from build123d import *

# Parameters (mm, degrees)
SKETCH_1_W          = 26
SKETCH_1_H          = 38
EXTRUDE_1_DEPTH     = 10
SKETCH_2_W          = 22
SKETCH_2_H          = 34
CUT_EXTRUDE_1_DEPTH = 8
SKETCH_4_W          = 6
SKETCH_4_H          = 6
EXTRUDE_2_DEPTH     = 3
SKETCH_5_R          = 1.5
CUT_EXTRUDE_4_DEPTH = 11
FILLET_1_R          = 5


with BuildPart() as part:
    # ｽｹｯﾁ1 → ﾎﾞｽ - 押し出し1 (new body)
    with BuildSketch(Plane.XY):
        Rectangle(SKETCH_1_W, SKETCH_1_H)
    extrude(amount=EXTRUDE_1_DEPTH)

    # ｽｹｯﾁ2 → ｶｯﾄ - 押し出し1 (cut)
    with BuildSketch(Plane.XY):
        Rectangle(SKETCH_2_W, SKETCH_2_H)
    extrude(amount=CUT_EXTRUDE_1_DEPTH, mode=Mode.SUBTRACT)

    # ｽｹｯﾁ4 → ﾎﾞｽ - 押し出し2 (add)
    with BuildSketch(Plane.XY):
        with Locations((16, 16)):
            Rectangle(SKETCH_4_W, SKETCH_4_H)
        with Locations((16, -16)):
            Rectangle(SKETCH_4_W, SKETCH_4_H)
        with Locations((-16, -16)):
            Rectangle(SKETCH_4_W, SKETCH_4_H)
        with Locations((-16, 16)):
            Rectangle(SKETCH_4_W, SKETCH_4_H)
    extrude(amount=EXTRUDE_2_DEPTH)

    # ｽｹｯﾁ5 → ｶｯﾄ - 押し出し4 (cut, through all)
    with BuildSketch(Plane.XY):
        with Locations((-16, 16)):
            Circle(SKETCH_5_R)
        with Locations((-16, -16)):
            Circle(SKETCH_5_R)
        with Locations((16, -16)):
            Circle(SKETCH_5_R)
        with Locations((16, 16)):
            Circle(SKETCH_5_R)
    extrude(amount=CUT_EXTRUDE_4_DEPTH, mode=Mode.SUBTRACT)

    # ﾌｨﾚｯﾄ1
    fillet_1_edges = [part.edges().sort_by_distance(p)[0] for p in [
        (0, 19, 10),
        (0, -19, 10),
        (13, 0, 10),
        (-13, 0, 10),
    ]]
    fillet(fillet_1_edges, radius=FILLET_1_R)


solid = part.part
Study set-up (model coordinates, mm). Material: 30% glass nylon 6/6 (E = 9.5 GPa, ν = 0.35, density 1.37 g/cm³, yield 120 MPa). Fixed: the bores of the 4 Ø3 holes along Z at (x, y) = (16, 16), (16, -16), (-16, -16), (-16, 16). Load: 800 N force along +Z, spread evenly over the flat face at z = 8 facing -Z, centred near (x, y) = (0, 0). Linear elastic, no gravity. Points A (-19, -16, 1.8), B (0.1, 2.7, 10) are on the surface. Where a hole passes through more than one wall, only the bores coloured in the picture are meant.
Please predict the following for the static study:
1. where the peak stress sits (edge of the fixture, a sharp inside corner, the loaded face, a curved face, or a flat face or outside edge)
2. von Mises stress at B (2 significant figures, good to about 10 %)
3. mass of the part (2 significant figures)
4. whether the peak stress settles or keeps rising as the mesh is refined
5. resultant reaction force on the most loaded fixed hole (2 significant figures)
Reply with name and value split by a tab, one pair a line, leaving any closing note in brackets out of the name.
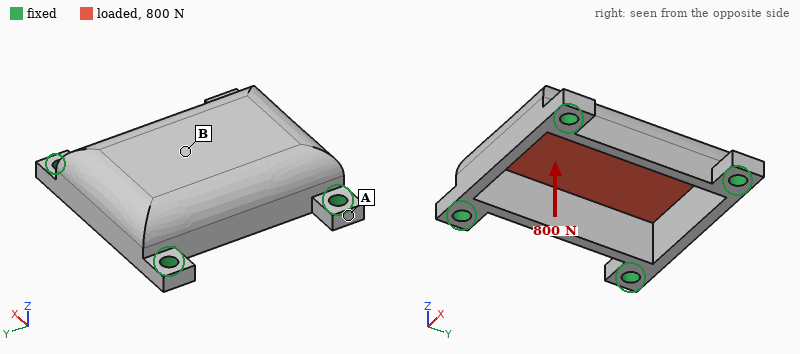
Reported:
where the peak stress sits	edge of the fixture
von Mises stress at B	53 MPa
mass of the part	4.9 g
whether the peak stress settles or keeps rising as the mesh is refined	keeps rising
resultant reaction force on the most loaded fixed hole	250 N
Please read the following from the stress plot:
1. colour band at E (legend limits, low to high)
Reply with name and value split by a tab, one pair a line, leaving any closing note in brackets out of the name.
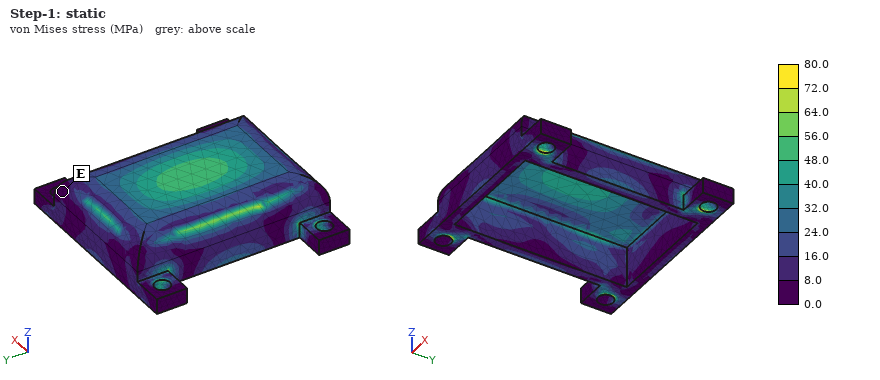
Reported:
colour band at E	0.0 to 8.0 MPa
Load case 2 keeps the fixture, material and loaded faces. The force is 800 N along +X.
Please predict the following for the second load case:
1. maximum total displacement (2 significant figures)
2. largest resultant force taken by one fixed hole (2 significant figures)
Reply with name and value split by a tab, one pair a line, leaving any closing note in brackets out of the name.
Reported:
maximum total displacement	85 µm
largest resultant force taken by one fixed hole	220 N
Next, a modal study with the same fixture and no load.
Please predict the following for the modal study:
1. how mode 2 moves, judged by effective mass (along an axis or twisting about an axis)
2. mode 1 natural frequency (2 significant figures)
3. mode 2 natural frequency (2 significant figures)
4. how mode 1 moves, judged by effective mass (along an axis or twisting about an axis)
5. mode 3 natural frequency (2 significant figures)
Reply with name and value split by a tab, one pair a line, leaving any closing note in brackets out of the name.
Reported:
how mode 2 moves, judged by effective mass	along X
mode 1 natural frequency	6800 Hz
mode 2 natural frequency	8800 Hz
how mode 1 moves, judged by effective mass	along Z
mode 3 natural frequency	9700 Hz
